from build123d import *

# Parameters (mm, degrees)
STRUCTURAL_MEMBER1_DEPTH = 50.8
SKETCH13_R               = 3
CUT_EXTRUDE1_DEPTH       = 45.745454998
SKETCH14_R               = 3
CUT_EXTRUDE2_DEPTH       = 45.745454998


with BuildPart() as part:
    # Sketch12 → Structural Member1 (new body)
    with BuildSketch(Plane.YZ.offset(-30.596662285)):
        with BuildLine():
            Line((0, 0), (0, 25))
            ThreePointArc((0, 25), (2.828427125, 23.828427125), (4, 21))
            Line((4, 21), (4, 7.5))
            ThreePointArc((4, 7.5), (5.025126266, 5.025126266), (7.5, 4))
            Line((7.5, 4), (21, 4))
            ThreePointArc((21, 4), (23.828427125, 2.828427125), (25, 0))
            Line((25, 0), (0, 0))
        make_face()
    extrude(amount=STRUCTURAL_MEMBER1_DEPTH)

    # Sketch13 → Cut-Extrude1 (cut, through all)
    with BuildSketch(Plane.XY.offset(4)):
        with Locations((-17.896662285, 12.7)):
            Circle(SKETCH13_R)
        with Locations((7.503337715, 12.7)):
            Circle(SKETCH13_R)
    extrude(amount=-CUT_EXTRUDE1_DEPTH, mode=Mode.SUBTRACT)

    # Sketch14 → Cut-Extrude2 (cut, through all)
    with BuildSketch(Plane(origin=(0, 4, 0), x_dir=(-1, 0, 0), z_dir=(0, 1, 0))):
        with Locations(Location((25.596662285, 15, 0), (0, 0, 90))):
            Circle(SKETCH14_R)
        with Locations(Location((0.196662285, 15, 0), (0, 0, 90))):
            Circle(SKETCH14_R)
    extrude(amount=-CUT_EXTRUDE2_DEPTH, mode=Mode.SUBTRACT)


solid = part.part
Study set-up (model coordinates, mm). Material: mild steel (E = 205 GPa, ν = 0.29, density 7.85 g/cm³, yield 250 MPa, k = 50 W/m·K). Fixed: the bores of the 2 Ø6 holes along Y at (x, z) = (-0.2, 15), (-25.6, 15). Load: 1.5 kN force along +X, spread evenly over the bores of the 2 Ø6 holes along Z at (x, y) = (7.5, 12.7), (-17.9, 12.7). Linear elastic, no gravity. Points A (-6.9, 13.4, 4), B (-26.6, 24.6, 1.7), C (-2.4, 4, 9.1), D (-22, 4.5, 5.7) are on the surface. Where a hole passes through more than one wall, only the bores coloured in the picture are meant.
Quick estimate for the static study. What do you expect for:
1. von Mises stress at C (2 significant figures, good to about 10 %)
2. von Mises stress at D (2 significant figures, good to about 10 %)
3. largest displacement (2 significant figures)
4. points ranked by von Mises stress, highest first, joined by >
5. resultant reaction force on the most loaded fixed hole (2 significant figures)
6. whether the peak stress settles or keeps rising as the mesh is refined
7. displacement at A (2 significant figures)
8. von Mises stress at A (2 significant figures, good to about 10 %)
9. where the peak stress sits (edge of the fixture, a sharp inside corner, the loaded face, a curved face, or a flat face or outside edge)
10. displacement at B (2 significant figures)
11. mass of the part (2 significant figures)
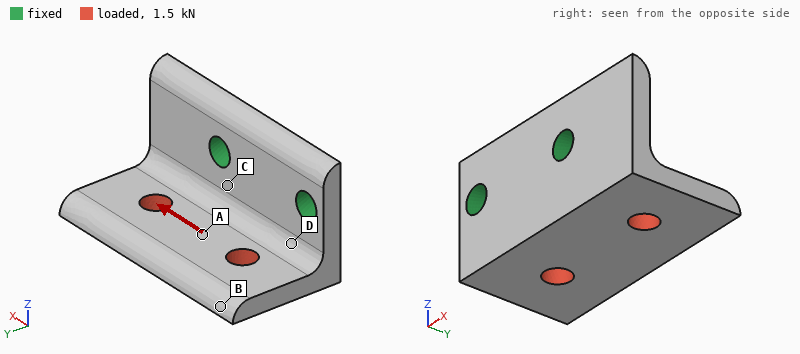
49 MPa
67 MPa
26 µm
D > C > A > B
1.2 kN
keeps rising
9.1 µm
23 MPa
edge of the fixture
18 µm
68 g
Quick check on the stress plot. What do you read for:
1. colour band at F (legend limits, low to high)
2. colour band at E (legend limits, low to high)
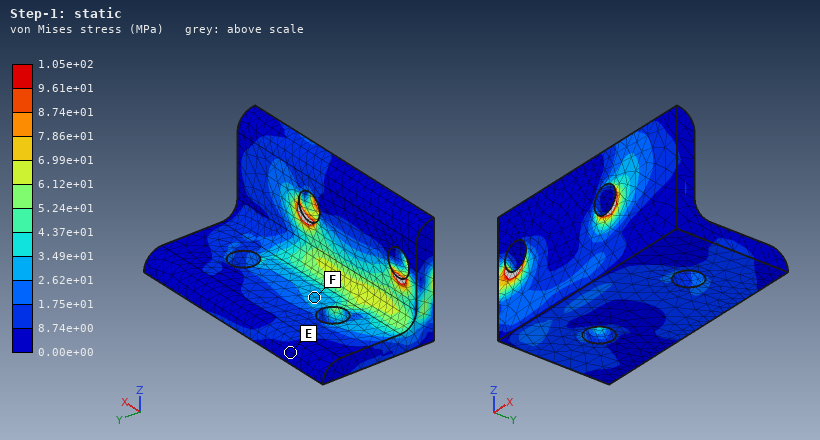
2.62e+01 to 3.49e+01 MPa
0.00e+00 to 8.74e+00 MPa
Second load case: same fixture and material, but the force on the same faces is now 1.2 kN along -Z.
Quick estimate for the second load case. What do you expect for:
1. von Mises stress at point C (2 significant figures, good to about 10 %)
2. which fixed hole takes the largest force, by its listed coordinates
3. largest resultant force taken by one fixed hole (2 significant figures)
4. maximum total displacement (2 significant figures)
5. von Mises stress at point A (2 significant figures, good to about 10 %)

120 MPa
(-0.2, 15)
900 N
76 µm
16 MPa
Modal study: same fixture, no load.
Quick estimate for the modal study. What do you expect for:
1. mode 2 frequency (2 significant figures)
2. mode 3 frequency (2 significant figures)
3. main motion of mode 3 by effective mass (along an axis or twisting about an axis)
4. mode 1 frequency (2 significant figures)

5900 Hz
8800 Hz
along Y
3700 Hz
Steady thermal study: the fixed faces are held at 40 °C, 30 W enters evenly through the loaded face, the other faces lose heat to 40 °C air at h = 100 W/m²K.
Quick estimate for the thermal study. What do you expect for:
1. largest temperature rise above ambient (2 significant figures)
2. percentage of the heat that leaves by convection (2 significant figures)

55 K
40 %
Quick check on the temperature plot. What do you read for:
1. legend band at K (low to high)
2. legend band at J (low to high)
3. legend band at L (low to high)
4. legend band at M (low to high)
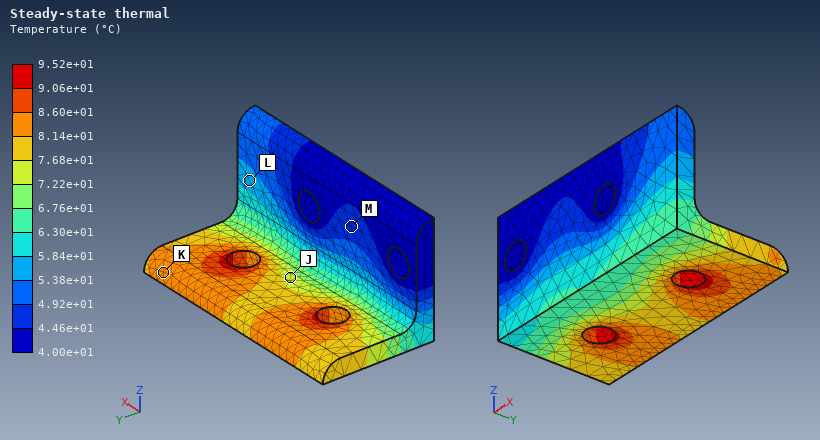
8.14e+01 to 8.60e+01 °C
7.22e+01 to 7.68e+01 °C
5.38e+01 to 5.84e+01 °C
4.46e+01 to 4.92e+01 °C
